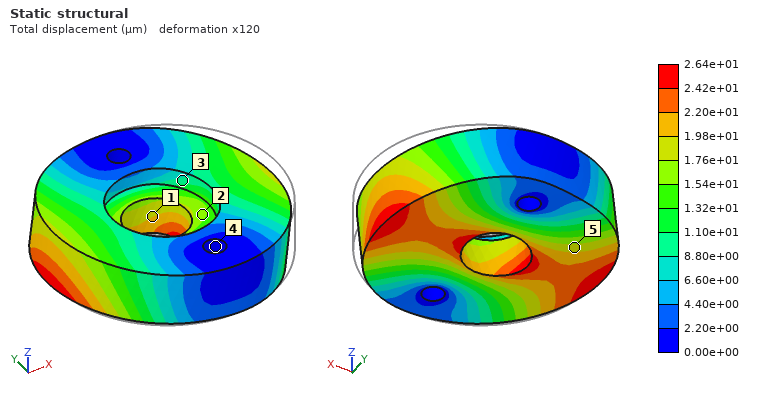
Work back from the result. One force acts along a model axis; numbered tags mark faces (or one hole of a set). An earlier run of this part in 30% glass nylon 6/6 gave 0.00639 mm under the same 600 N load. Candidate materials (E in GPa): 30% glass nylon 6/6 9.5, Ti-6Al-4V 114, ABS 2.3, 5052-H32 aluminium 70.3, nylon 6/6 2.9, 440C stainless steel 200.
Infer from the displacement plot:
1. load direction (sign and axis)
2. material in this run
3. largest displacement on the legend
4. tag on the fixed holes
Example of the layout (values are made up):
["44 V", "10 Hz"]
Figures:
["-X", "ABS", "2.64e+01 µm", "4"]
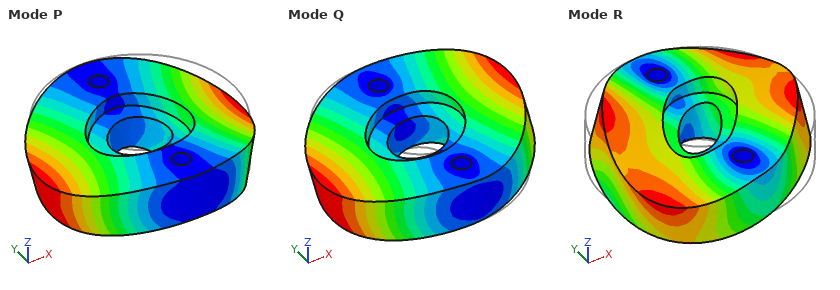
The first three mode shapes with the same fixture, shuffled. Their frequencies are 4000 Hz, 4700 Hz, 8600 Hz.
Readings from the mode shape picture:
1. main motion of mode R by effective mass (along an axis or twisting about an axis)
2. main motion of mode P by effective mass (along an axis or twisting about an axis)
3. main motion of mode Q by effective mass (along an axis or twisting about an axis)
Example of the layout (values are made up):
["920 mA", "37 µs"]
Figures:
["twisting about Z", "along Z", "twisting about Y"]
